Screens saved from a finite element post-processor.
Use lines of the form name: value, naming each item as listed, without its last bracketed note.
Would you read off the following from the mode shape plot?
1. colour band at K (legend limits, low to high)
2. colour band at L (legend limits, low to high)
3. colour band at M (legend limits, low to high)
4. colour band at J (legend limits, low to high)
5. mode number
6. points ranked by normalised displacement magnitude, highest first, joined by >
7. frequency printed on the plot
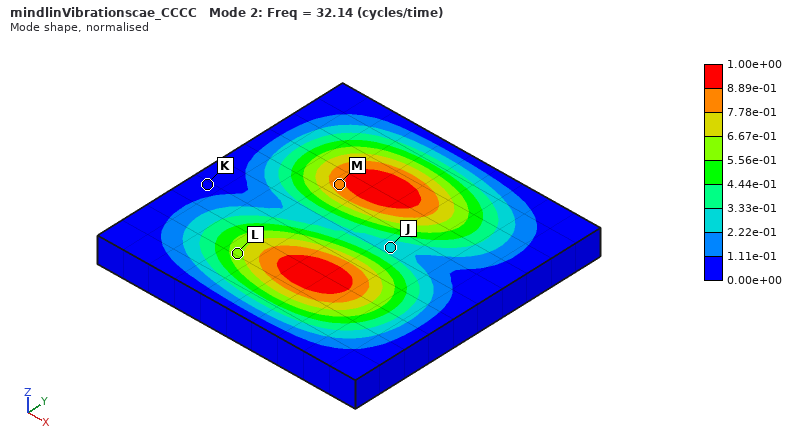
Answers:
colour band at K: 0.00e+00 to 1.11e-01
colour band at L: 5.56e-01 to 6.67e-01
colour band at M: 7.78e-01 to 8.89e-01
colour band at J: 2.22e-01 to 3.33e-01
mode number: 2
points ranked by normalised displacement magnitude, highest first, joined by >: M > L > J > K
frequency printed on the plot: 32.14
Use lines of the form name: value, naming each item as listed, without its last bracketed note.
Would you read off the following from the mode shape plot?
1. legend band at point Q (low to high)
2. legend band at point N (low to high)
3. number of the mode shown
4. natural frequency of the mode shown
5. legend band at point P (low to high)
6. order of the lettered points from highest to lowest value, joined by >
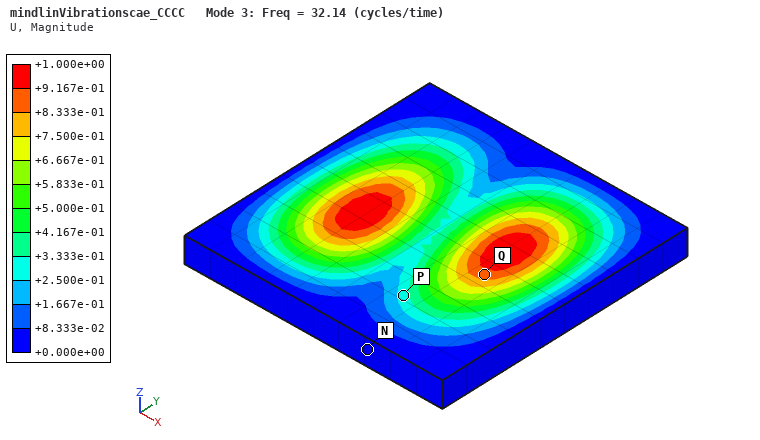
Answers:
legend band at point Q: +8.333e-01 to +9.167e-01
legend band at point N: +0.000e+00 to +8.333e-02
number of the mode shown: 3
natural frequency of the mode shown: 32.14
legend band at point P: +2.500e-01 to +3.333e-01
order of the lettered points from highest to lowest value, joined by >: Q > P > N
